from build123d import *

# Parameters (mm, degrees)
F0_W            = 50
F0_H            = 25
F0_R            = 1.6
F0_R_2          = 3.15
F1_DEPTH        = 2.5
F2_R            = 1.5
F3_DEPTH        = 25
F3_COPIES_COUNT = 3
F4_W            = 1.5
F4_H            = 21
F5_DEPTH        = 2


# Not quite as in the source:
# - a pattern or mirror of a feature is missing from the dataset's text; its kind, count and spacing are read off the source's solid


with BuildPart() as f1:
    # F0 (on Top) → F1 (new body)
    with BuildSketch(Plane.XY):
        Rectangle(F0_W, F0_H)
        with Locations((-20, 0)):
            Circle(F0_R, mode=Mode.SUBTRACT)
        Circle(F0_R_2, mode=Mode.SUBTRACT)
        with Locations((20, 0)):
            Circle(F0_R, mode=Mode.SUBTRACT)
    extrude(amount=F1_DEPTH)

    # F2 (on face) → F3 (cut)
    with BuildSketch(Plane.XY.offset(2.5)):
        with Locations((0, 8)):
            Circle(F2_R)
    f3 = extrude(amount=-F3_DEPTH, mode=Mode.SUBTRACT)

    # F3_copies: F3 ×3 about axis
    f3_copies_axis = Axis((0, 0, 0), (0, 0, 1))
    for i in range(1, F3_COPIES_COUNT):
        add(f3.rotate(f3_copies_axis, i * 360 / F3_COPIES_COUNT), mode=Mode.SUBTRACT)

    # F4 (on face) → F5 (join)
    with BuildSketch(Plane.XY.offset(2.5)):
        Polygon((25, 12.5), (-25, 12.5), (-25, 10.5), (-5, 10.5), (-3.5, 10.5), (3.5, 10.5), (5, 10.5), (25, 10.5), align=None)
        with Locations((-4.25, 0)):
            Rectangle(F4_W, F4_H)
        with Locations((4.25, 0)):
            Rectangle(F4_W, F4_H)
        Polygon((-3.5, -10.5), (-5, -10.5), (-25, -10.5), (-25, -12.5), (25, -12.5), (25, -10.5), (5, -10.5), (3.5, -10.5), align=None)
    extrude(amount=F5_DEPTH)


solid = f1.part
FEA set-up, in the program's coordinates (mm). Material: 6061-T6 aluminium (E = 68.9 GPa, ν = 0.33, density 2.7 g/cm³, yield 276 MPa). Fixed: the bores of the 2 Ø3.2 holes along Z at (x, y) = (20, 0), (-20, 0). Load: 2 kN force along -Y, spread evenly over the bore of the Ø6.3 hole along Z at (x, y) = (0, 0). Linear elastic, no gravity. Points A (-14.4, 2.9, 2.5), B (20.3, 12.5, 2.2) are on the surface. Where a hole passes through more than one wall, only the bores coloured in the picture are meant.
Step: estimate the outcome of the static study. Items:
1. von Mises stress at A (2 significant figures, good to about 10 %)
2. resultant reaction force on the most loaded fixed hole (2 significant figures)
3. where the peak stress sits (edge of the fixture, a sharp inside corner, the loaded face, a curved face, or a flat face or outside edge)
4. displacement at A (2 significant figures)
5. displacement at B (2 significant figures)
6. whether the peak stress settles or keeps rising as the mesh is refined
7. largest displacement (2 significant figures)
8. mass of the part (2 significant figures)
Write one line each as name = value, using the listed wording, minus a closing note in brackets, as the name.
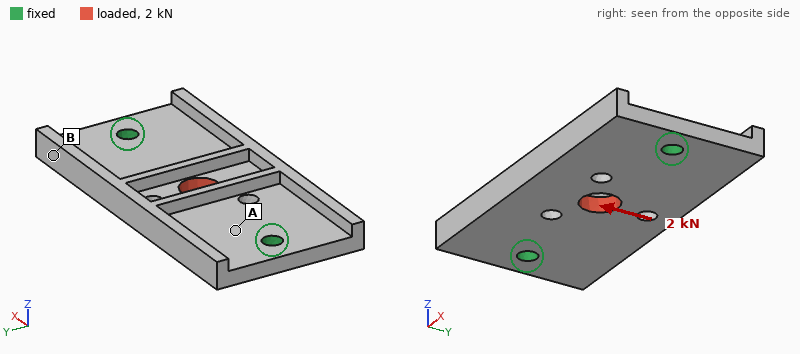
von Mises stress at A = 45 MPa
resultant reaction force on the most loaded fixed hole = 1.0 kN
where the peak stress sits = edge of the fixture
displacement at A = 8.5 µm
displacement at B = 8.3 µm
whether the peak stress settles or keeps rising as the mesh is refined = keeps rising
largest displacement = 29 µm
mass of the part = 9.4 g
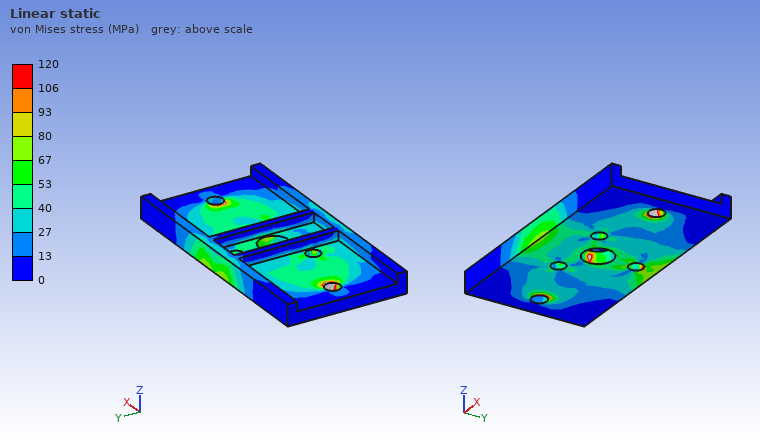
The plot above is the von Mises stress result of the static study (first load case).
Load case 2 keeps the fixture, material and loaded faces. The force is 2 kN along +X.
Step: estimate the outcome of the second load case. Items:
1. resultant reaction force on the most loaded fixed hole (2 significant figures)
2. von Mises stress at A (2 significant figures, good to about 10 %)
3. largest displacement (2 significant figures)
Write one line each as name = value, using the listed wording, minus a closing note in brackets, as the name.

resultant reaction force on the most loaded fixed hole = 1.0 kN
von Mises stress at A = 33 MPa
largest displacement = 10 µm
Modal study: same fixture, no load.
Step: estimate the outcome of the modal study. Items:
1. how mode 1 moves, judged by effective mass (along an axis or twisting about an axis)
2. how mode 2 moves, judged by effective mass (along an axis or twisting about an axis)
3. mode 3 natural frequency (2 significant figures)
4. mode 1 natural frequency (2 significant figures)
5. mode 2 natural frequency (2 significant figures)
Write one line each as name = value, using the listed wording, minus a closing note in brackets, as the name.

how mode 1 moves, judged by effective mass = twisting about X
how mode 2 moves, judged by effective mass = along Z
mode 3 natural frequency = 12 kHz
mode 1 natural frequency = 6300 Hz
mode 2 natural frequency = 7100 Hz
